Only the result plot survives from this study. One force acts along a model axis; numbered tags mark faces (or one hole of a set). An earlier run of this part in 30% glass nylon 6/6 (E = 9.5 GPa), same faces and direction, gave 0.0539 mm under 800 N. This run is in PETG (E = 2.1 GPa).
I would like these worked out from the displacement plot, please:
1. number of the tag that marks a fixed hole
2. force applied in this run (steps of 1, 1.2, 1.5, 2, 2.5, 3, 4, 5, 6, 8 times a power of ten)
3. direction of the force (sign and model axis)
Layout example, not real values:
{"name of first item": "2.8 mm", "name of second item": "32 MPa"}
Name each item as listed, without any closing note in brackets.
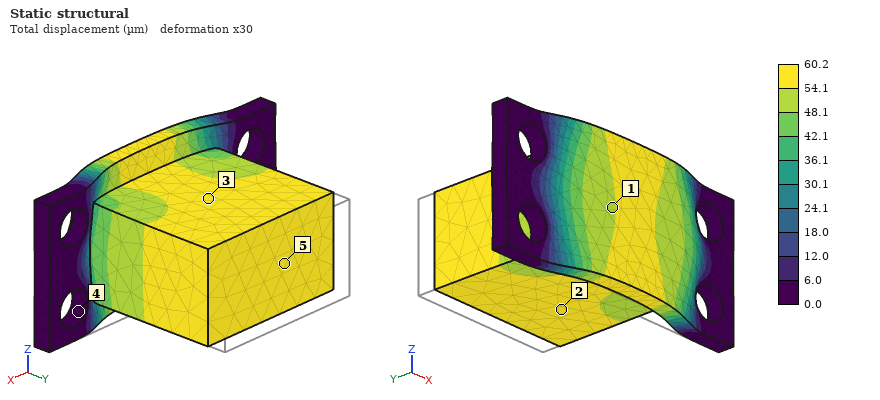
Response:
{"number of the tag that marks a fixed hole": "4", "force applied in this run": "200 N", "direction of the force": "-Y"}
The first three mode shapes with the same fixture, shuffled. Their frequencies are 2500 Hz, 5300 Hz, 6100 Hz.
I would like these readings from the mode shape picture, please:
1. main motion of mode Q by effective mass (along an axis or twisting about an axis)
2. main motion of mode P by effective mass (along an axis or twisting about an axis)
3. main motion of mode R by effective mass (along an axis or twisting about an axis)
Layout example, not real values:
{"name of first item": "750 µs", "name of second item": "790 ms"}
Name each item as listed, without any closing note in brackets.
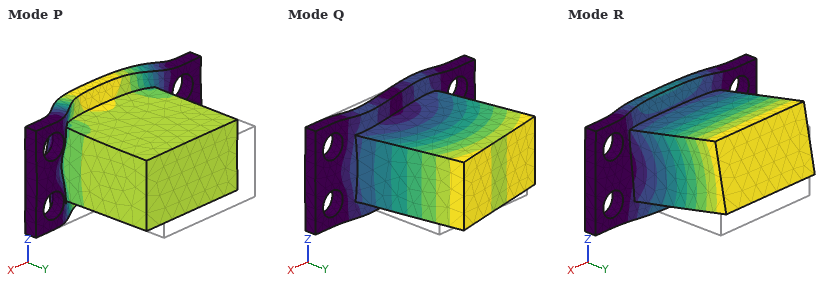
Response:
{"main motion of mode Q by effective mass": "along X", "main motion of mode P by effective mass": "along Y", "main motion of mode R by effective mass": "along Z"}
